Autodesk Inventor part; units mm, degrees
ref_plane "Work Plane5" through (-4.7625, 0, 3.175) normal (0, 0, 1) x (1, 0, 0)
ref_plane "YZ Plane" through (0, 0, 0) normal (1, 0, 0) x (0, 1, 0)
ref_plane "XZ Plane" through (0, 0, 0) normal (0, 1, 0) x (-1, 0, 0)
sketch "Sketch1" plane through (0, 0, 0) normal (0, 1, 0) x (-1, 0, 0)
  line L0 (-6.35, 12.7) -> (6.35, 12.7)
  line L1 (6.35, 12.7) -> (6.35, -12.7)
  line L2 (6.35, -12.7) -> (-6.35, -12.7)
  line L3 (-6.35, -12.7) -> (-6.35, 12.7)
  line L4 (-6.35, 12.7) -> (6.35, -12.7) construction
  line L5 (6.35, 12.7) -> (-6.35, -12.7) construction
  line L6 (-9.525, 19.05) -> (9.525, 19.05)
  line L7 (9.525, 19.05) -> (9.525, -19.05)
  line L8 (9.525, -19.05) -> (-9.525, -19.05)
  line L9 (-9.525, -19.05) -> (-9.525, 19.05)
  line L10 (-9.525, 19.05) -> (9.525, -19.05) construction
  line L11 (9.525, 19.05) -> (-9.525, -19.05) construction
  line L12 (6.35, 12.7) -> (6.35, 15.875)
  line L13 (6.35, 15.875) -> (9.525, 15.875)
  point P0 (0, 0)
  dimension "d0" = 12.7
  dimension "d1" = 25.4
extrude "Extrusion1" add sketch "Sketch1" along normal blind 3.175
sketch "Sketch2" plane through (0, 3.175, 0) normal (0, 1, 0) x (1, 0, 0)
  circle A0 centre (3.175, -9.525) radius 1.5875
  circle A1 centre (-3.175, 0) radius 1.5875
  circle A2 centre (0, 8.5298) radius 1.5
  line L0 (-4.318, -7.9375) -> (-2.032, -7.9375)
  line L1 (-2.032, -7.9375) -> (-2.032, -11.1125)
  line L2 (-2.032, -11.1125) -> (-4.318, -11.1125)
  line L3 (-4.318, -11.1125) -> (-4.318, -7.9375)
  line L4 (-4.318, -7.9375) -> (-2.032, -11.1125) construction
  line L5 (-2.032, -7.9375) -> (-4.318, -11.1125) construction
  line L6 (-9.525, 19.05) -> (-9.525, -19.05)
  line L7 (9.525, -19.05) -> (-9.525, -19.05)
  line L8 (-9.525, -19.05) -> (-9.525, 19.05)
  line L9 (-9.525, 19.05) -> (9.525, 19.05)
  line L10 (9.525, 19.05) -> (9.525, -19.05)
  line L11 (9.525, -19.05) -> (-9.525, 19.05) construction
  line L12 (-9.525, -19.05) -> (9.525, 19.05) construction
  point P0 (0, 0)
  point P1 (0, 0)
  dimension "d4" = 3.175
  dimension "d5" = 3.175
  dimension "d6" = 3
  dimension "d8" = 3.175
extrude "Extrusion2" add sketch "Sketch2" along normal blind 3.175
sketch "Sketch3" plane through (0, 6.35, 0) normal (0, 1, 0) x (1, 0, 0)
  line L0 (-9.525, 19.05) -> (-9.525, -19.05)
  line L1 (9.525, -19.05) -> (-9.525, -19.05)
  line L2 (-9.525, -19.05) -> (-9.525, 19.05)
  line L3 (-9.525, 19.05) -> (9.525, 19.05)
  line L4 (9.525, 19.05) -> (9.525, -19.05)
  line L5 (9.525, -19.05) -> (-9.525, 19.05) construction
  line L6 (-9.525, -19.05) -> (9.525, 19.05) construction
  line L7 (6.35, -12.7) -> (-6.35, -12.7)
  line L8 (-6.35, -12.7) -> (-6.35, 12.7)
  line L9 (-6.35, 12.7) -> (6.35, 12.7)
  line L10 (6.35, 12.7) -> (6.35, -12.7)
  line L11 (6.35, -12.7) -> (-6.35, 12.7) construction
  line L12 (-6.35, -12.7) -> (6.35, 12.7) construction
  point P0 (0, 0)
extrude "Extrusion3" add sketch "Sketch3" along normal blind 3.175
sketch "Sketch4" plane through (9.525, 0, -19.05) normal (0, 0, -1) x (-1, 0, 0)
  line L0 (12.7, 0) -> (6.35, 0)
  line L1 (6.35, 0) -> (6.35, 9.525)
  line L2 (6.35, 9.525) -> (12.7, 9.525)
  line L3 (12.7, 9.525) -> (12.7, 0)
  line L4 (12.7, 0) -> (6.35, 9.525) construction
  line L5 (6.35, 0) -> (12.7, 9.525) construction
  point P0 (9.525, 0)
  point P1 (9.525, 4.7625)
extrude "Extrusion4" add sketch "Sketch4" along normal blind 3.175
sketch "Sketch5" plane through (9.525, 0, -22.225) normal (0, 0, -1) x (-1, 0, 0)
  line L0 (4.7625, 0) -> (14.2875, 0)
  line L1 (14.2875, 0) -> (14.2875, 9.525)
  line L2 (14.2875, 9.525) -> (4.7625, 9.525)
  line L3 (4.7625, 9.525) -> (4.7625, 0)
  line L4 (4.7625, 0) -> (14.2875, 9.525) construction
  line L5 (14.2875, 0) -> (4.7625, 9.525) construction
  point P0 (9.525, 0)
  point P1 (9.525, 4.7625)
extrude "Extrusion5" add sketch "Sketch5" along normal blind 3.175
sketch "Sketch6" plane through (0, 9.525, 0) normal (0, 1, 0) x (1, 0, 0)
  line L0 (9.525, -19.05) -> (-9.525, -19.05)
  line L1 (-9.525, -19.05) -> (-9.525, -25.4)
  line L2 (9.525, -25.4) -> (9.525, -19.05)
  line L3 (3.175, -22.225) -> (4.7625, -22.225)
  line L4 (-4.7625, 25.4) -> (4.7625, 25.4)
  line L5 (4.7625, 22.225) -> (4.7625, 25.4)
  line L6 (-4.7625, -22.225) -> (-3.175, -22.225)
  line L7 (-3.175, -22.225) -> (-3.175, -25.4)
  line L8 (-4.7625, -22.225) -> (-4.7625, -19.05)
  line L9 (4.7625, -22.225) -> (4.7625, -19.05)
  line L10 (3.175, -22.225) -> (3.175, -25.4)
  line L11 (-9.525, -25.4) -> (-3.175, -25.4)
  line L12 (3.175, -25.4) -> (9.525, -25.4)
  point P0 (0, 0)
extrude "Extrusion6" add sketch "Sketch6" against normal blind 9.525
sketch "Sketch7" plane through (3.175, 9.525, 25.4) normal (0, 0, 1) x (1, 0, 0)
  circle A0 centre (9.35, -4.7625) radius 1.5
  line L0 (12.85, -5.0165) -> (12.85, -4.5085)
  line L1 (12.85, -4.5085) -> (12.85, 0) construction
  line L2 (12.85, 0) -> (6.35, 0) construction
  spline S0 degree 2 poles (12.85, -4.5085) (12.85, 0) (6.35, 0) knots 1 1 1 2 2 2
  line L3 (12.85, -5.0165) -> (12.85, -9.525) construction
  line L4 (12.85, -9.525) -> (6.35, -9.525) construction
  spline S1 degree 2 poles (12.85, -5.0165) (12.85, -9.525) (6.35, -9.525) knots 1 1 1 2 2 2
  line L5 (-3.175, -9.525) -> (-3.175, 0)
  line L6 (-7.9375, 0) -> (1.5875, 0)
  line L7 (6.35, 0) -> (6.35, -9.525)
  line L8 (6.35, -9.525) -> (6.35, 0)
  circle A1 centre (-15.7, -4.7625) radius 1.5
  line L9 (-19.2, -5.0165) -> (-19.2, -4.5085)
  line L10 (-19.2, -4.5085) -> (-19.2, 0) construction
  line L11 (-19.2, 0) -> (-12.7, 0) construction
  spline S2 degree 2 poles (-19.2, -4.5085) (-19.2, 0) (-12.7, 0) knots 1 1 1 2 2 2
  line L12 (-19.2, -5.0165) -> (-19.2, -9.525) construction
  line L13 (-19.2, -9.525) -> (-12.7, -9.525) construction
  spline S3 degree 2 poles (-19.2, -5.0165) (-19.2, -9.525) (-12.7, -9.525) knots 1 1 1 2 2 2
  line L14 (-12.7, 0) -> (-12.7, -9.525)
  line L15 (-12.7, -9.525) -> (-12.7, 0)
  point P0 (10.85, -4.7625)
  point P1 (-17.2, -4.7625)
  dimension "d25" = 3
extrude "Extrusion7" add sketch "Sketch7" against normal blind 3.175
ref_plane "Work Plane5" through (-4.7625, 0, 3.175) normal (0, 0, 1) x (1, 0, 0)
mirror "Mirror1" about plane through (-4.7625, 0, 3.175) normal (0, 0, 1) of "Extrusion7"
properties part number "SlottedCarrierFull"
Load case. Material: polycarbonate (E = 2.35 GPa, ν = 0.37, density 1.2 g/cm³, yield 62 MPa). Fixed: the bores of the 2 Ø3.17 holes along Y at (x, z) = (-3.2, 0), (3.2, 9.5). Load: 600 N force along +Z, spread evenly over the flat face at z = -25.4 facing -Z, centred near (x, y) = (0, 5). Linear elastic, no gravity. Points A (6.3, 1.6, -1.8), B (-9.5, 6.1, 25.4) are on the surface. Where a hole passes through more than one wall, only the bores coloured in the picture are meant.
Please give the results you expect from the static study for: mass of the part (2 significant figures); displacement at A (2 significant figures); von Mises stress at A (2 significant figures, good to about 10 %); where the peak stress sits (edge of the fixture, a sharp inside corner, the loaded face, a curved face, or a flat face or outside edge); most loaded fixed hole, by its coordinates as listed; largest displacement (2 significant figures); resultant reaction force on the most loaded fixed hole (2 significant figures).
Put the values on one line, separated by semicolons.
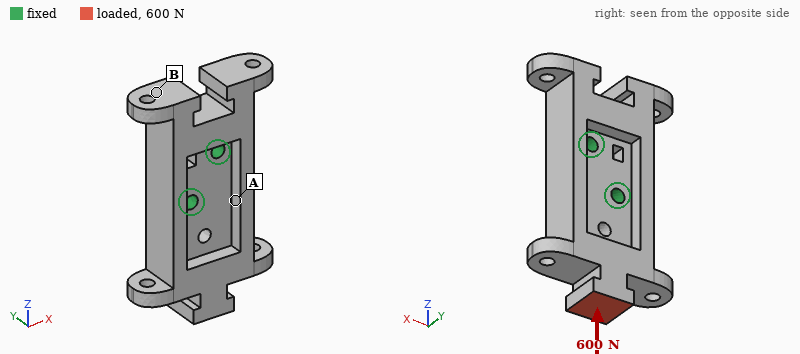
7.8 g; 0.039 mm; 4.7 MPa; a curved face; (-3.2, 0); 0.14 mm; 340 N
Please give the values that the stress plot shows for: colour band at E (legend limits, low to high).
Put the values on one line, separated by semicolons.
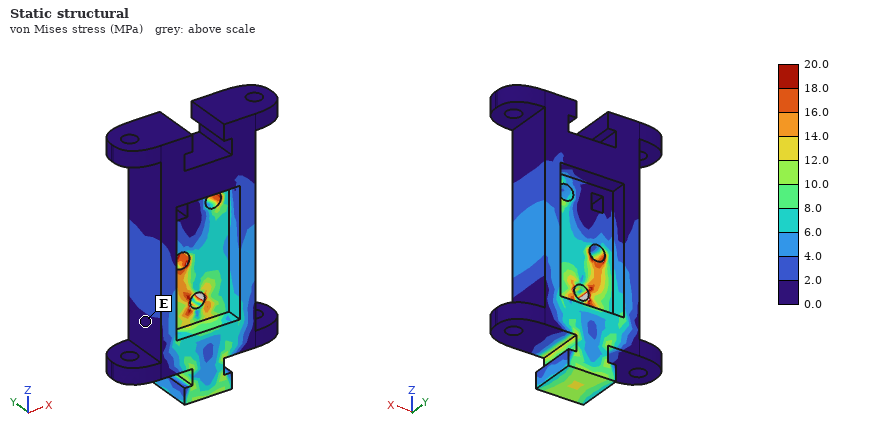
0.0 to 2.0 MPa
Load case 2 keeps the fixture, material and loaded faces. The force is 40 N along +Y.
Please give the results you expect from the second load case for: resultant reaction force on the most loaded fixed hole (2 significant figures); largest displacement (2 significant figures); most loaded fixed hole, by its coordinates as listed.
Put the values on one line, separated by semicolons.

78 N; 0.47 mm; (-3.2, 0)
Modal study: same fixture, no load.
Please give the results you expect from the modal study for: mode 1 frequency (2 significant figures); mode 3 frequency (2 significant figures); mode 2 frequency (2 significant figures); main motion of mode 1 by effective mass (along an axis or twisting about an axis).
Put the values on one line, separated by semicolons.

1300 Hz; 2600 Hz; 2500 Hz; along Y
